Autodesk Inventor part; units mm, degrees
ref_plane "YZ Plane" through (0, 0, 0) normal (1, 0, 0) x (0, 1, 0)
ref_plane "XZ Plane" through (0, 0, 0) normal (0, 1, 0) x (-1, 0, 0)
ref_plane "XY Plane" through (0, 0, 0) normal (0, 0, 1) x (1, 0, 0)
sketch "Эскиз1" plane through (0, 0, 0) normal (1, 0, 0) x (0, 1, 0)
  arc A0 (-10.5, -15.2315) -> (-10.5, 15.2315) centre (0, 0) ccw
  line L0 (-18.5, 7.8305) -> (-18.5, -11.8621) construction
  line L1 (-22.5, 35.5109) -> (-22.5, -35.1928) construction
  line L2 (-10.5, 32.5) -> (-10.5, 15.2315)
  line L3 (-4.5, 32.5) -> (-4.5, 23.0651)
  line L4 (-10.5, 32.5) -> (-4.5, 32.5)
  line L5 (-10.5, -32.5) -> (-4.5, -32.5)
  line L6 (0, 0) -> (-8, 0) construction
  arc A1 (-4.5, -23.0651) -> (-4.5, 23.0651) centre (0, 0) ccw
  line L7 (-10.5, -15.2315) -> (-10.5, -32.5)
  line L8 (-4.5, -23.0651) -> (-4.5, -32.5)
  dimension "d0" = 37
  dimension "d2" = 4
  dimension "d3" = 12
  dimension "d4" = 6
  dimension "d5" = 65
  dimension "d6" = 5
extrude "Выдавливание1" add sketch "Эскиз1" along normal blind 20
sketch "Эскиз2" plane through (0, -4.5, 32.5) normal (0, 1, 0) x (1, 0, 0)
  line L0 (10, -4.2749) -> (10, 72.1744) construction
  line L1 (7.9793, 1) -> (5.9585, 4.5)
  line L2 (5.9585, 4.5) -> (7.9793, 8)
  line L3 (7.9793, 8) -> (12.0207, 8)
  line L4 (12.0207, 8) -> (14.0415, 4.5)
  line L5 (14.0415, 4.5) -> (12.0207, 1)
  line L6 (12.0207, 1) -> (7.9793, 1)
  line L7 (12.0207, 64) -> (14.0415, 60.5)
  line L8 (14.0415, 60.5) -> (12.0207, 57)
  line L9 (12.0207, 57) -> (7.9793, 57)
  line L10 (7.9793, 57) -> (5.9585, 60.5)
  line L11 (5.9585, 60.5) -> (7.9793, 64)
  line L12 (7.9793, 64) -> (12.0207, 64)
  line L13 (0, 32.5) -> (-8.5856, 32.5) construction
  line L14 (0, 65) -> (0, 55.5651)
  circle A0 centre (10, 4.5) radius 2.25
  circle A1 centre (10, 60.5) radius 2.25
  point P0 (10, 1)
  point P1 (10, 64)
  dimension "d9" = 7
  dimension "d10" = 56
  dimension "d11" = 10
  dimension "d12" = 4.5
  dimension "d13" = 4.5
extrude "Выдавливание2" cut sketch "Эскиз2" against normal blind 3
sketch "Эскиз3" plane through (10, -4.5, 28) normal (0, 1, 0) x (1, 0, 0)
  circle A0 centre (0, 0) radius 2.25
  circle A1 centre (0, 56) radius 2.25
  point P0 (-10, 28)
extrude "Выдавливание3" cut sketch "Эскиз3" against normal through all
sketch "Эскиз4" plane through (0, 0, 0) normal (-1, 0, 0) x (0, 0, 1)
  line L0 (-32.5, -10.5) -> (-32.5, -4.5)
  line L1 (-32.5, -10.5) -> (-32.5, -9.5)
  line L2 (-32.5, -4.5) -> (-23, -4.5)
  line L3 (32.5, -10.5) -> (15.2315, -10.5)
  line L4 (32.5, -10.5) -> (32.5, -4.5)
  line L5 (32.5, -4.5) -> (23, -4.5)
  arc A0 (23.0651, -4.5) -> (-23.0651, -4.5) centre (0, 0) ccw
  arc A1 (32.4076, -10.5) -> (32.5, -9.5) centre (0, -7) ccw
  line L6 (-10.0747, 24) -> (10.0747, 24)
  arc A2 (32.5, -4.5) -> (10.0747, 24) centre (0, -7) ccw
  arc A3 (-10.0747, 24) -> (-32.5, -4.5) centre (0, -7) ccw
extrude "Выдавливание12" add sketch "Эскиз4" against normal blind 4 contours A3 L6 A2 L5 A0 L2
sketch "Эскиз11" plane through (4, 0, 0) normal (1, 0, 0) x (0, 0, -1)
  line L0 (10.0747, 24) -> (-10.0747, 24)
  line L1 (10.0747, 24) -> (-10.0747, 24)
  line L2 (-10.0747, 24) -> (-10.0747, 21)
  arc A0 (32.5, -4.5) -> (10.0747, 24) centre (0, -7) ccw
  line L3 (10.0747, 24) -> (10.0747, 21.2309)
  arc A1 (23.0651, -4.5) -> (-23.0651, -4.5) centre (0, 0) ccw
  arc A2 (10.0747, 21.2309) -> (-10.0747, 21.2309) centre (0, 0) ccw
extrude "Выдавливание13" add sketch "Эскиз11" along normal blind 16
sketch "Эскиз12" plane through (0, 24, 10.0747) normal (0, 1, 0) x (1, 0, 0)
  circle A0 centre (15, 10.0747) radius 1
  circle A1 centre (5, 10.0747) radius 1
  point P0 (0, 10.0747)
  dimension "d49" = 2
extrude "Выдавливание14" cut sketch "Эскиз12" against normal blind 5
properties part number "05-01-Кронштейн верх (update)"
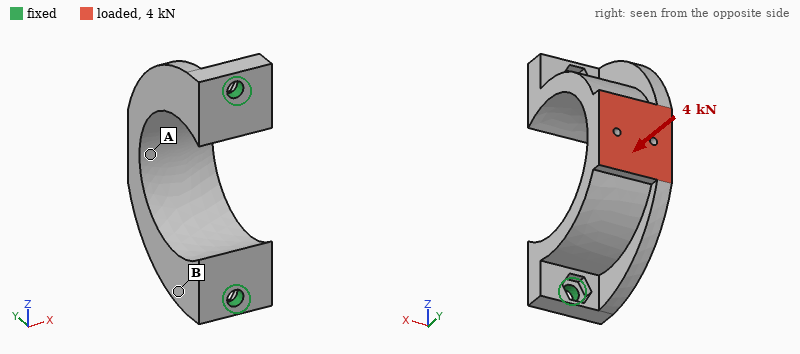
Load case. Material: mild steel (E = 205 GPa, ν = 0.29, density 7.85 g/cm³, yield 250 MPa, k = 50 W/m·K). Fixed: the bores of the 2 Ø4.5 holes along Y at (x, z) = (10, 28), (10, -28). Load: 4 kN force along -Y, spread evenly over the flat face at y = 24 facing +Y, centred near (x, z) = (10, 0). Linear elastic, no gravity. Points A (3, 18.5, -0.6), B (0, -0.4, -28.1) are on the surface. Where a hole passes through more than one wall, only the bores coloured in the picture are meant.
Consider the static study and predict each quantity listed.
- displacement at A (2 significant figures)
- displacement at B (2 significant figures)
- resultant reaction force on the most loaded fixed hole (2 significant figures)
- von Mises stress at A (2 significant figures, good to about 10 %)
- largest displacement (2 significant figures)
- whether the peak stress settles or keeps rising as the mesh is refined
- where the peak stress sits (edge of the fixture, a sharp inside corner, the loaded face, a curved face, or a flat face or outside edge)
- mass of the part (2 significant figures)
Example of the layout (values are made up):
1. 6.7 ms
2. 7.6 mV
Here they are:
1. 16 µm
2. 3.6 µm
3. 2.3 kN
4. 68 MPa
5. 21 µm
6. keeps rising
7. edge of the fixture
8. 100 g
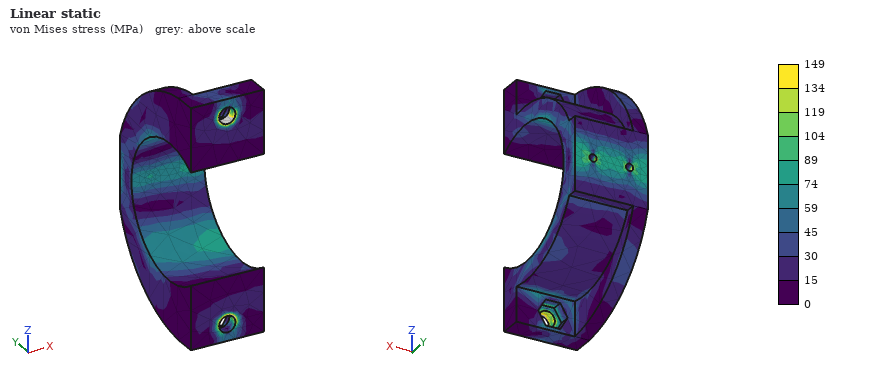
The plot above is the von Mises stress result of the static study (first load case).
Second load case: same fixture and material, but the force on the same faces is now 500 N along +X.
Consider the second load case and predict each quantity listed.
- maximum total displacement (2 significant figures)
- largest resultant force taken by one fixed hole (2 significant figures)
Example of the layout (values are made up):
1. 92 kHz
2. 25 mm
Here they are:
1. 50 µm
2. 250 N
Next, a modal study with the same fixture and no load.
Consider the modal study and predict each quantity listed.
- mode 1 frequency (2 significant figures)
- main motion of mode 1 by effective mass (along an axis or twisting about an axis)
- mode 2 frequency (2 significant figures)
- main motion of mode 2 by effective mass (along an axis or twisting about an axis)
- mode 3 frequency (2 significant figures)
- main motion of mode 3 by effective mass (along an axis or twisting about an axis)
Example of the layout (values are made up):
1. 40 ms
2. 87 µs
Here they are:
1. 2800 Hz
2. along X
3. 5600 Hz
4. along Z
5. 7700 Hz
6. twisting about Y
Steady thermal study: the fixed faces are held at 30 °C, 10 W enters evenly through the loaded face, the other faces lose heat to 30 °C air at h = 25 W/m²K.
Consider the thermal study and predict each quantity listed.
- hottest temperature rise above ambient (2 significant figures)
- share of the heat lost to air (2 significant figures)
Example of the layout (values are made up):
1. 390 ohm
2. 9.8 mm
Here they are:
1. 33 K
2. 22 %
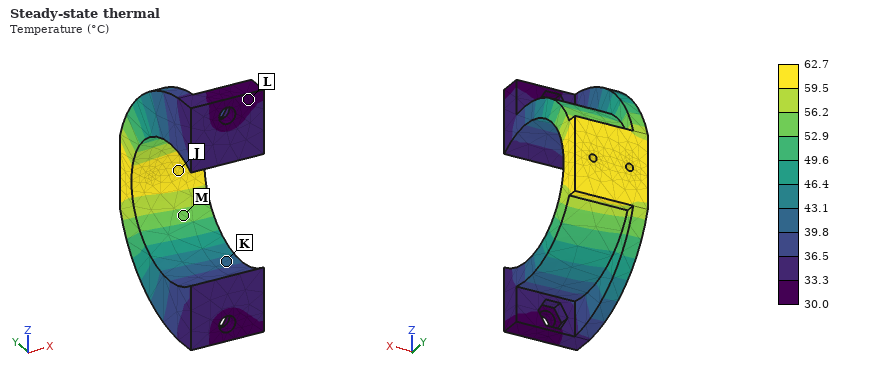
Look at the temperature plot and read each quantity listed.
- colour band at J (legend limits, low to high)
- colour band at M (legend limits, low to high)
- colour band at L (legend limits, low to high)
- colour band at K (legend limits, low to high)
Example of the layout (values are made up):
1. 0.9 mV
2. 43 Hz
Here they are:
1. 59.5 to 62.7 °C
2. 52.9 to 56.2 °C
3. 30.0 to 33.3 °C
4. 39.8 to 43.1 °C
